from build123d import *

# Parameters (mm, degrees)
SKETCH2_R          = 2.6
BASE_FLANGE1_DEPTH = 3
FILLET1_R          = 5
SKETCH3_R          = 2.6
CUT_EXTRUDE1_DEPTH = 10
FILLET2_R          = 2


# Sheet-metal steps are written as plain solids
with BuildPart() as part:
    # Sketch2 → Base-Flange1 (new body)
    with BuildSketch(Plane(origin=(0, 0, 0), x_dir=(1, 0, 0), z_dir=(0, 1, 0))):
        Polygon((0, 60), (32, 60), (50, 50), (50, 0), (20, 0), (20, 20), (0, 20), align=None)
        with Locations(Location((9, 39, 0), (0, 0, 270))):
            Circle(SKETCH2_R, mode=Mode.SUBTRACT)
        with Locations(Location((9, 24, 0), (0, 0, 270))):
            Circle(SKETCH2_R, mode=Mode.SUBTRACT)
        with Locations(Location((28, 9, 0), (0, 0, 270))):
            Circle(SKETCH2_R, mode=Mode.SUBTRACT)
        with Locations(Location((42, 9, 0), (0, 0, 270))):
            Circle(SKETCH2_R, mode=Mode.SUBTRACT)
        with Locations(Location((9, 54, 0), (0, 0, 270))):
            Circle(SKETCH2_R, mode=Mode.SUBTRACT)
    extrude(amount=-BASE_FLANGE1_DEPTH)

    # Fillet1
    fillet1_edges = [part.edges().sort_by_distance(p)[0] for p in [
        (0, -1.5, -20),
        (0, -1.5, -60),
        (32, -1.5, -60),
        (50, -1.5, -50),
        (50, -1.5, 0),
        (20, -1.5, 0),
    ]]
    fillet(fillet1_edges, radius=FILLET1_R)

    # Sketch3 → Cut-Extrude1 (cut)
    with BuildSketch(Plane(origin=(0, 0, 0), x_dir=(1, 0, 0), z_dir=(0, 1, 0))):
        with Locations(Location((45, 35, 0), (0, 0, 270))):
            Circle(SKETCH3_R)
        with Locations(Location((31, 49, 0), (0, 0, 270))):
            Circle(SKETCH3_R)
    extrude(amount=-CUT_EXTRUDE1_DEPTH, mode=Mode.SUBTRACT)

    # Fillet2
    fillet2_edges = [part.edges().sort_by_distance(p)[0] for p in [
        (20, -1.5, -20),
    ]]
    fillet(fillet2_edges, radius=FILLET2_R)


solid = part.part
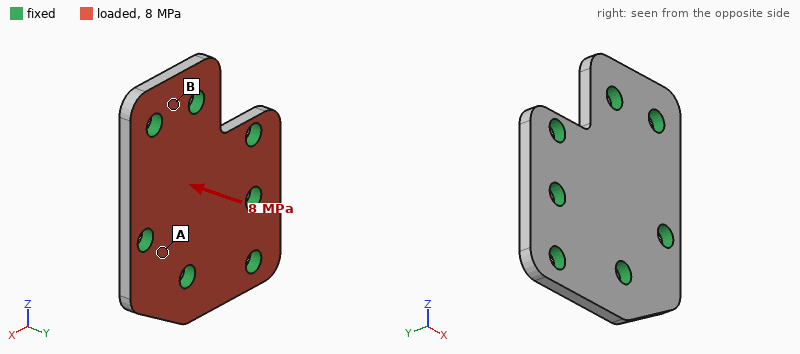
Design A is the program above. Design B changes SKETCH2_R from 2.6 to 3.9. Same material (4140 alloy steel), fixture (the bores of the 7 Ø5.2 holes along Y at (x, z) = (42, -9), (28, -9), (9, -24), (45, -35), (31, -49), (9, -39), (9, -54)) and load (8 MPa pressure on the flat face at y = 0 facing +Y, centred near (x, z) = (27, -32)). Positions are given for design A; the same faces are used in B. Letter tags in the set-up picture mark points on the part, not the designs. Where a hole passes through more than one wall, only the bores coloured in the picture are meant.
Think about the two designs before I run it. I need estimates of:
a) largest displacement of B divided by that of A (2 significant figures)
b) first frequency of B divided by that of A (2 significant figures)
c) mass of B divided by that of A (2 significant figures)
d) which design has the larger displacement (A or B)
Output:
0.91
1.1
0.94
A
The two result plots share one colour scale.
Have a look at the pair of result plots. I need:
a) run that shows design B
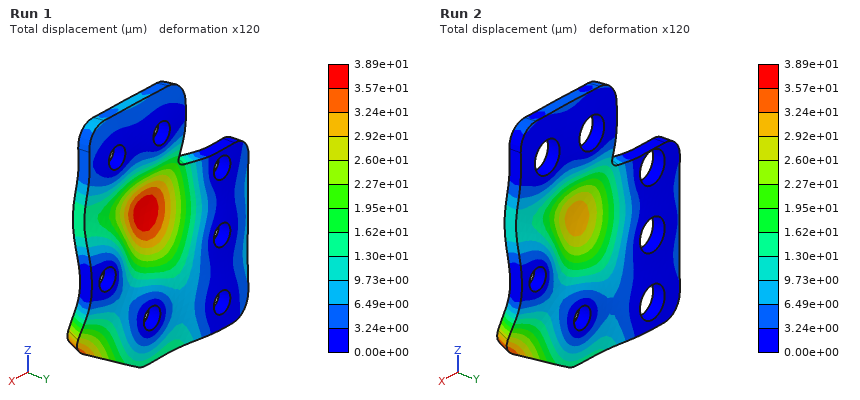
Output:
Run 2
